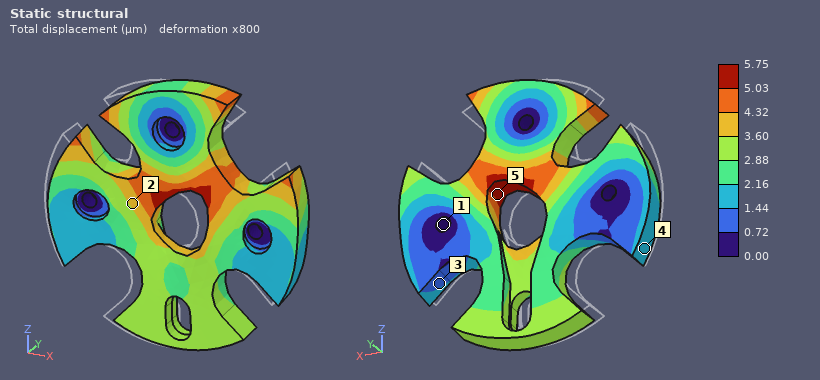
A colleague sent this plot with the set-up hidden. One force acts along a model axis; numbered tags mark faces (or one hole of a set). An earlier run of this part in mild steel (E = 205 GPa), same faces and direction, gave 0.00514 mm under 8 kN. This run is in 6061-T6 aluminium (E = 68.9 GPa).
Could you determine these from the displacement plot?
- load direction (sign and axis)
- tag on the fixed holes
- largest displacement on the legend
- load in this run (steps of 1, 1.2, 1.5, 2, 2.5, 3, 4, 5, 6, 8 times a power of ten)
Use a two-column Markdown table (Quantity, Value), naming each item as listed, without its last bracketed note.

| Quantity | Value |
|---|---|
| load direction | +X |
| tag on the fixed holes | 1 |
| largest displacement on the legend | 5.75 µm |
| load in this run | 3 kN |
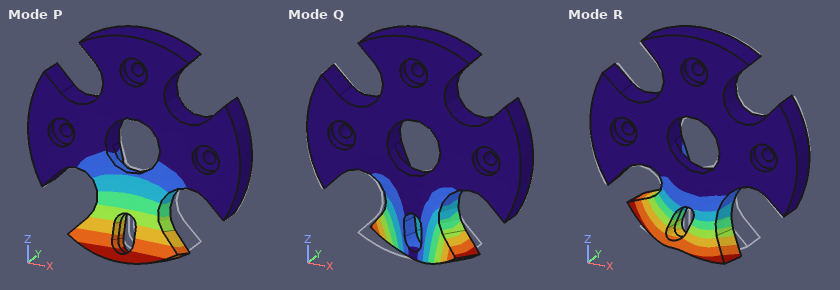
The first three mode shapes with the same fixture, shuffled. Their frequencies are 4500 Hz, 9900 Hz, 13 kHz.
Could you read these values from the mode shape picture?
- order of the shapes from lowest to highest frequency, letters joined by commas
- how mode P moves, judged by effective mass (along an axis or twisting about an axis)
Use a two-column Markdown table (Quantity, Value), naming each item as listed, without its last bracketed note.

| Quantity | Value |
|---|---|
| order of the shapes from lowest to highest frequency, letters joined by commas | P, Q, R |
| how mode P moves, judged by effective mass | along Y |
